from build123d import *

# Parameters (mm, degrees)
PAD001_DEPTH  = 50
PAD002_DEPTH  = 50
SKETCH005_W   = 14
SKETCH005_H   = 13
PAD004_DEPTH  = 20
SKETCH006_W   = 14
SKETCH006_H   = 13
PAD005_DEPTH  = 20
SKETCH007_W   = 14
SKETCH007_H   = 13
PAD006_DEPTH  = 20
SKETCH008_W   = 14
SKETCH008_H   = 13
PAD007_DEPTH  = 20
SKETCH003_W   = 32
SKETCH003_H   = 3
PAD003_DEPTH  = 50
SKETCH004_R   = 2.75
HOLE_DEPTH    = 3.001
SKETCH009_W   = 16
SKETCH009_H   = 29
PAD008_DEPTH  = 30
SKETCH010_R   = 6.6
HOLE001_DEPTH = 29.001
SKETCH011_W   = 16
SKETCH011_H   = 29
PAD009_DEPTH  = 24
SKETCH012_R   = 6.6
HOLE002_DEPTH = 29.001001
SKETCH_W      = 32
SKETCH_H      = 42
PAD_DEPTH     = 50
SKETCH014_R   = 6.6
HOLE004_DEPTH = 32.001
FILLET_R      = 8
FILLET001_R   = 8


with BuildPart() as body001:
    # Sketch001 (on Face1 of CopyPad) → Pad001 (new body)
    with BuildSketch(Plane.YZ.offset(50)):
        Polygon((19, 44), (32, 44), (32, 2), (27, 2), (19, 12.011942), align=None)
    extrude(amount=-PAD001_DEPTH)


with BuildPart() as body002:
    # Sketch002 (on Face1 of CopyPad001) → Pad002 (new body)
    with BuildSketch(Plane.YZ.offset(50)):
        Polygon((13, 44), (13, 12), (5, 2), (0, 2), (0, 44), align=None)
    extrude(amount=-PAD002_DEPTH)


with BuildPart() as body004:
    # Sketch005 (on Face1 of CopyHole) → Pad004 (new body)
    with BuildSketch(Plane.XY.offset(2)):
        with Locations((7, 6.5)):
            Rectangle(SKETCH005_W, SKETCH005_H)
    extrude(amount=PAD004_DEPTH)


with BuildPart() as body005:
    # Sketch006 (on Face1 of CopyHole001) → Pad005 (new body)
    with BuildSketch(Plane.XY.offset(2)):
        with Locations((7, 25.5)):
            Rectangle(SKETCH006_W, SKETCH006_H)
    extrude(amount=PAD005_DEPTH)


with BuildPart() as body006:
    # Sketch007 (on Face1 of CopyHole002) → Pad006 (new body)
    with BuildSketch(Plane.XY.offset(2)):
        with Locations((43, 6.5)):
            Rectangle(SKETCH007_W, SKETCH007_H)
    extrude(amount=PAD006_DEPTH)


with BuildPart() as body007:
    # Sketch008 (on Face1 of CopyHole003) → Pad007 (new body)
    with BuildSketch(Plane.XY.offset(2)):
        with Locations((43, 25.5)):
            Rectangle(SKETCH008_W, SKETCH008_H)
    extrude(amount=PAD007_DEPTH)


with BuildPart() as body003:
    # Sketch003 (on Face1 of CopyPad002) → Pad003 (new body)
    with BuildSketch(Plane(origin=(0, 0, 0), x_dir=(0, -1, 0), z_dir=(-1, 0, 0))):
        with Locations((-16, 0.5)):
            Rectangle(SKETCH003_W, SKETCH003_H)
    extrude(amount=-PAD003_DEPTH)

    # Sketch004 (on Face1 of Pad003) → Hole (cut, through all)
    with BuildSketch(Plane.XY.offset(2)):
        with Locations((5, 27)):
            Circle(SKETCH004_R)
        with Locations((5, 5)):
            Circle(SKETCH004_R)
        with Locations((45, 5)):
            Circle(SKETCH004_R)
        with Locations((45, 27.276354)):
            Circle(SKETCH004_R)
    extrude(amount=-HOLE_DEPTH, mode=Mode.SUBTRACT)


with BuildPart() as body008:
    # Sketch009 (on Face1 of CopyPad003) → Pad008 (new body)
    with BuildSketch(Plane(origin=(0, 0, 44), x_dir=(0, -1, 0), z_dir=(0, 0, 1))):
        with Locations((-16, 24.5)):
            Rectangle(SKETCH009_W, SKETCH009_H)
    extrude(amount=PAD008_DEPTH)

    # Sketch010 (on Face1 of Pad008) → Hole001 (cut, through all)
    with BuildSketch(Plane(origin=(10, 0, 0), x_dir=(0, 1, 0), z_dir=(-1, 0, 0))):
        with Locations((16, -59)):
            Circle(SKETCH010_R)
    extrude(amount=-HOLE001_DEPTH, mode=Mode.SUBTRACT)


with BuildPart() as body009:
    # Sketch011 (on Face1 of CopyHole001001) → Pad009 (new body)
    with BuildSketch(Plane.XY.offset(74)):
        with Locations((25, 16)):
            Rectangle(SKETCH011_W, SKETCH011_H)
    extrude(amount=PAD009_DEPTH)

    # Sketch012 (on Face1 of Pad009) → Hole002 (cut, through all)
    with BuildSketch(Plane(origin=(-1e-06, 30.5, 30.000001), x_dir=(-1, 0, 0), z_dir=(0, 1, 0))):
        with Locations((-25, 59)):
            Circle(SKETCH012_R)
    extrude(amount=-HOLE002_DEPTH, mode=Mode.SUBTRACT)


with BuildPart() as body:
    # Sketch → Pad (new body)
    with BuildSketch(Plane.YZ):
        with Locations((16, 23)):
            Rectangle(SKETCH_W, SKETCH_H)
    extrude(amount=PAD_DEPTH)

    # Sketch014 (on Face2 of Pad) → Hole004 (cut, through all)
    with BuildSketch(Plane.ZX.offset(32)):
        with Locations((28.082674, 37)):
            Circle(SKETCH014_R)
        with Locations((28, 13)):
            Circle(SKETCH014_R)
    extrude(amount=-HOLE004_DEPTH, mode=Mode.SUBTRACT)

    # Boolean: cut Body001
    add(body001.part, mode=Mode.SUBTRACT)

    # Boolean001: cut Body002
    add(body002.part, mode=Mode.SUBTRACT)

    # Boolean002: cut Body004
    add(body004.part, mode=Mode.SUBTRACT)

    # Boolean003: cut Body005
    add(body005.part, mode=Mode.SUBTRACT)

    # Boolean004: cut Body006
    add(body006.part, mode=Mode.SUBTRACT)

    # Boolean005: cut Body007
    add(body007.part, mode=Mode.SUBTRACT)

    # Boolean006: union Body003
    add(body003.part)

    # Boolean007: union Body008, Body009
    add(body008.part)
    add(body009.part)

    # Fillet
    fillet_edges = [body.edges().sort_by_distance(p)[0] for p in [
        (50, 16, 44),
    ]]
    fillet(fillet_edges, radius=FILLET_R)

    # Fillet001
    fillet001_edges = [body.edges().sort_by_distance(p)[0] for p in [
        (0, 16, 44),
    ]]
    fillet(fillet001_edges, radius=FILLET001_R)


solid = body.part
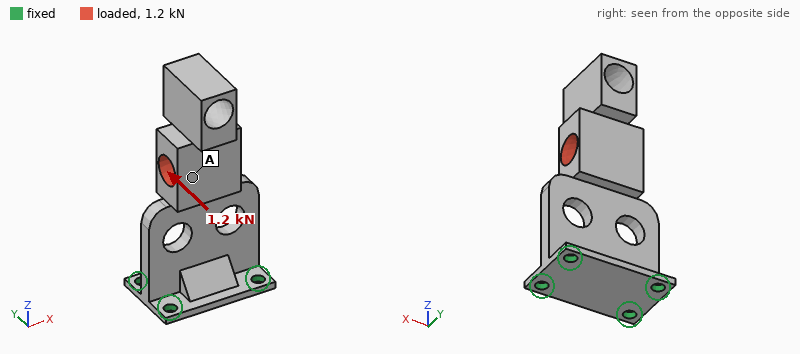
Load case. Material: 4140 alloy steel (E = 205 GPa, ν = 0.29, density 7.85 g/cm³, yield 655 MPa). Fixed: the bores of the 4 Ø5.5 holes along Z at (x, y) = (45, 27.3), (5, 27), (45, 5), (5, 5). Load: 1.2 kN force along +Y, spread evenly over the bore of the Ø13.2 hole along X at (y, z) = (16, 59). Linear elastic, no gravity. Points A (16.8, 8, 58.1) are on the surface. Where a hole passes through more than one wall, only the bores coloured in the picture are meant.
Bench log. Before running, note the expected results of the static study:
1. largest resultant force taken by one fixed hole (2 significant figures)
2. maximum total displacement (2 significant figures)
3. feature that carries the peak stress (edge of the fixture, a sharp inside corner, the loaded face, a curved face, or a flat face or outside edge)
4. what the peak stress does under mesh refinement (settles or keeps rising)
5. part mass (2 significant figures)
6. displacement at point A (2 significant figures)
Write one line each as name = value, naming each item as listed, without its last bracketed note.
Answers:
largest resultant force taken by one fixed hole = 2.0 kN
maximum total displacement = 1.1 mm
feature that carries the peak stress = edge of the fixture
what the peak stress does under mesh refinement = keeps rising
part mass = 270 g
displacement at point A = 0.52 mm
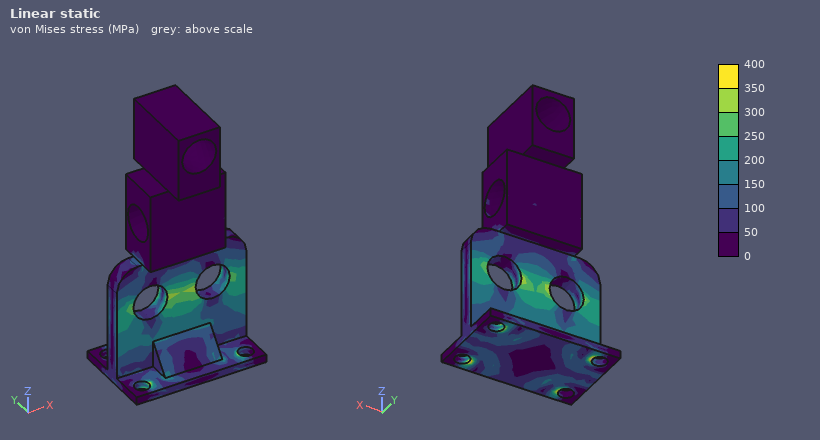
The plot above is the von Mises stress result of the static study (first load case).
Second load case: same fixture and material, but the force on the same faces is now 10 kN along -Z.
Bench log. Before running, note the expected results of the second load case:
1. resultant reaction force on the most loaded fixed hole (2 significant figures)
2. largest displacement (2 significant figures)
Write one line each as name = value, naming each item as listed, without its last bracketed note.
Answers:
resultant reaction force on the most loaded fixed hole = 2.7 kN
largest displacement = 37 µm
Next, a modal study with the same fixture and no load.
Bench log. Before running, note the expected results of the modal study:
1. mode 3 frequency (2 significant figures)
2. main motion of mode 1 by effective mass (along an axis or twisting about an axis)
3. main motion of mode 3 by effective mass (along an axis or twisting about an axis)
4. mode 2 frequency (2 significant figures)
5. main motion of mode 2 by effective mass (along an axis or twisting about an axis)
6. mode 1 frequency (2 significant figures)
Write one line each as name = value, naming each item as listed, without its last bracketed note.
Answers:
mode 3 frequency = 3200 Hz
main motion of mode 1 by effective mass = along Y
main motion of mode 3 by effective mass = twisting about Z
mode 2 frequency = 1900 Hz
main motion of mode 2 by effective mass = along X
mode 1 frequency = 480 Hz
